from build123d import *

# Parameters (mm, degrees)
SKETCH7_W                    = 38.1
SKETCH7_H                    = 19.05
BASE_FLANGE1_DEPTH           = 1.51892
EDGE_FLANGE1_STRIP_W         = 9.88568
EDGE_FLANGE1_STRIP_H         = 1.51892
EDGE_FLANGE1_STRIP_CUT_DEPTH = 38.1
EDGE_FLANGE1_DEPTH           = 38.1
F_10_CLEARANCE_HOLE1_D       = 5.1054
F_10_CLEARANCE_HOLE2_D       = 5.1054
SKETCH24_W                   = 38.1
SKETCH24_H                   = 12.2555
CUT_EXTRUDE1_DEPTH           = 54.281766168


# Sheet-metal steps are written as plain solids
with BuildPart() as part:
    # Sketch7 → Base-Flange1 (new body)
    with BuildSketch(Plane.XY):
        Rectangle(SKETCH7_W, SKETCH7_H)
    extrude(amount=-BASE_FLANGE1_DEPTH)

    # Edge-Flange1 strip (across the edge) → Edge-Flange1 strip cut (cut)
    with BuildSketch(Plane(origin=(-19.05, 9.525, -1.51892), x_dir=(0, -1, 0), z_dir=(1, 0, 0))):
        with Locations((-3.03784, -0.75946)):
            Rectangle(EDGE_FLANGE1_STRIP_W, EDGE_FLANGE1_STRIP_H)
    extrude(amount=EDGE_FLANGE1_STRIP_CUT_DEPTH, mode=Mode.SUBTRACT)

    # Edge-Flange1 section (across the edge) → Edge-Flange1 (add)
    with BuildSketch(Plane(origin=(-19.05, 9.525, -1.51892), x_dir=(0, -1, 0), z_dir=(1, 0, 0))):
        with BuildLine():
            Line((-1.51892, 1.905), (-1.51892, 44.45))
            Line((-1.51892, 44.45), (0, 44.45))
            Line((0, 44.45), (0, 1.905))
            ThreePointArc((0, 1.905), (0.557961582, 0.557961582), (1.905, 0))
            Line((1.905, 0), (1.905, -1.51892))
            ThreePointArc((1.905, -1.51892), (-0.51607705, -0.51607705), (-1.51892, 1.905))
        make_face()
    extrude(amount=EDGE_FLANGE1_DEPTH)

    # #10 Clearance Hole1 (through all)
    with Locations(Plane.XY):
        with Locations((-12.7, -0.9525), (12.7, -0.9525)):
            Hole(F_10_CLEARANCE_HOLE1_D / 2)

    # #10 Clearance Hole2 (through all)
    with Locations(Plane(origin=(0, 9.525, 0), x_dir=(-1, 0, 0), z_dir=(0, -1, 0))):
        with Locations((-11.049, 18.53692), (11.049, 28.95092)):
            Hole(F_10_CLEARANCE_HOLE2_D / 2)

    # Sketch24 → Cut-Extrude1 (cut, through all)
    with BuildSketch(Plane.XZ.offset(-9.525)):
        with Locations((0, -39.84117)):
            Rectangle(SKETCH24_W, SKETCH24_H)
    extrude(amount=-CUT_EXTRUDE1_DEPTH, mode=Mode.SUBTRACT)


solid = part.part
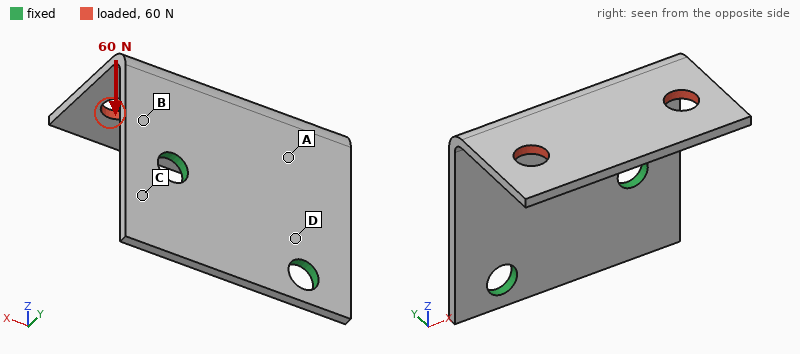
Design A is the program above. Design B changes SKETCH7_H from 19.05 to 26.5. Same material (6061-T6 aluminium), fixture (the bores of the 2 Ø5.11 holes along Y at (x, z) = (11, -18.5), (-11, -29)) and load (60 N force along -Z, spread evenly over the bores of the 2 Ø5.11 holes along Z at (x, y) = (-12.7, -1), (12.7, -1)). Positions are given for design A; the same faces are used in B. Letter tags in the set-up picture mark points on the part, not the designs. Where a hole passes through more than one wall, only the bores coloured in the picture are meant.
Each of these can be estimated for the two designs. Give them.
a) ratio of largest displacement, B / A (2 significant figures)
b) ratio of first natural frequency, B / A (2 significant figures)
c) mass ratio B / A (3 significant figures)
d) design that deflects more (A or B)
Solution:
1.1
0.84
1.08
B
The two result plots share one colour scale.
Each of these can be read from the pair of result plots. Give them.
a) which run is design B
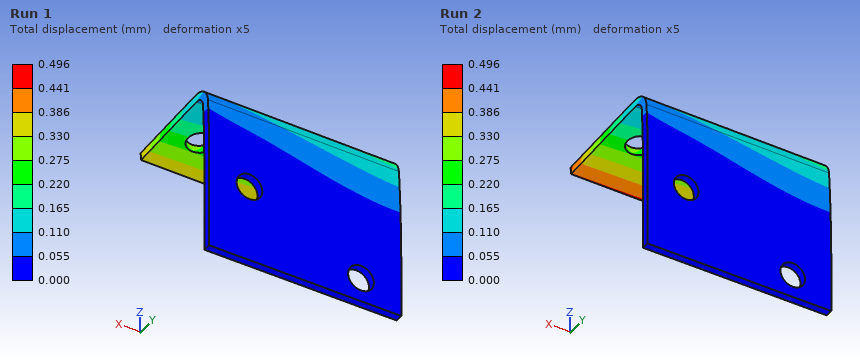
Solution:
Run 2
